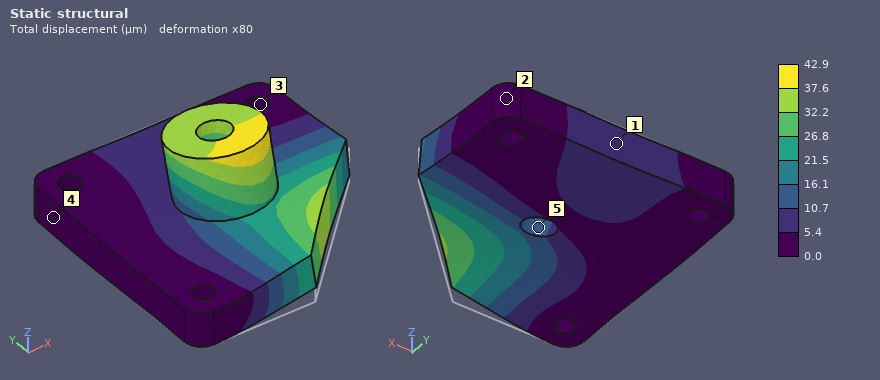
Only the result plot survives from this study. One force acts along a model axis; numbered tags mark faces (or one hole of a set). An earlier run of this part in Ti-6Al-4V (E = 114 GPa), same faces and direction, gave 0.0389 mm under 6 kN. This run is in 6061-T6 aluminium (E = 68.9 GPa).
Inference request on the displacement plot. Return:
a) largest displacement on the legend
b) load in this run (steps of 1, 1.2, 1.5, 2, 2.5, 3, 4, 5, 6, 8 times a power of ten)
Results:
42.9 µm
4 kN
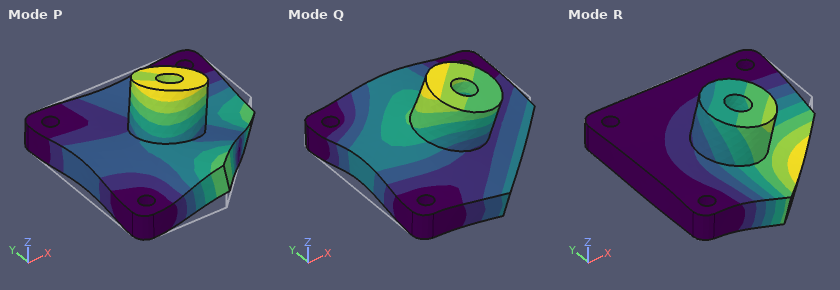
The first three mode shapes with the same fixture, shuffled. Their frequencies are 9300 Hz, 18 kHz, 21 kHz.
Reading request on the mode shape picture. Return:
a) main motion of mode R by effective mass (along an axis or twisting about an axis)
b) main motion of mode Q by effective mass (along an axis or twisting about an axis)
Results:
along Z
along Z
